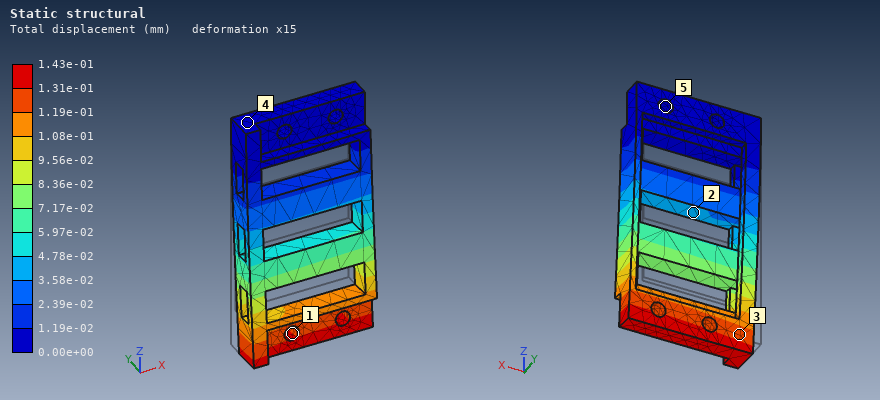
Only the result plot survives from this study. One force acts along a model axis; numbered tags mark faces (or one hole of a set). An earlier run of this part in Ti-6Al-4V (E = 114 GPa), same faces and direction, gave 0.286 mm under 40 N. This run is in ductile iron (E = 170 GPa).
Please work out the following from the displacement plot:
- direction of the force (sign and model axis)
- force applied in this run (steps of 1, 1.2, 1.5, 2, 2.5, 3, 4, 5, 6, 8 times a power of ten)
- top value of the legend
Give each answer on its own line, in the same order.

-Y
30 N
1.43e-01 mm
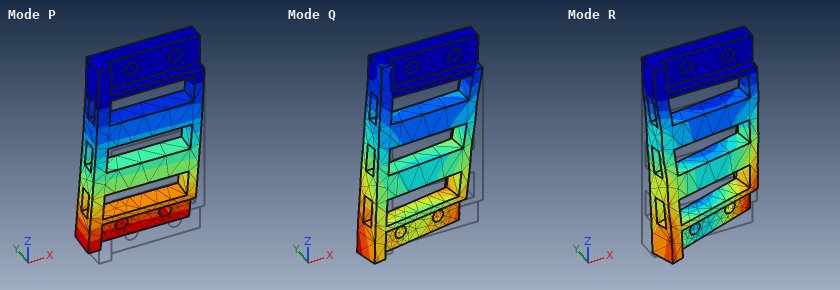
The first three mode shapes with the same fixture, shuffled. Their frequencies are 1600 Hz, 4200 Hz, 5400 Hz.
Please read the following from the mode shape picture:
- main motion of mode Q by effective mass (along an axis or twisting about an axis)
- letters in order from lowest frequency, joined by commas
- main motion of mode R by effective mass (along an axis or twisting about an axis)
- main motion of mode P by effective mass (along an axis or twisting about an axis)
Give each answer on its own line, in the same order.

along X
P, Q, R
along X
along Y
